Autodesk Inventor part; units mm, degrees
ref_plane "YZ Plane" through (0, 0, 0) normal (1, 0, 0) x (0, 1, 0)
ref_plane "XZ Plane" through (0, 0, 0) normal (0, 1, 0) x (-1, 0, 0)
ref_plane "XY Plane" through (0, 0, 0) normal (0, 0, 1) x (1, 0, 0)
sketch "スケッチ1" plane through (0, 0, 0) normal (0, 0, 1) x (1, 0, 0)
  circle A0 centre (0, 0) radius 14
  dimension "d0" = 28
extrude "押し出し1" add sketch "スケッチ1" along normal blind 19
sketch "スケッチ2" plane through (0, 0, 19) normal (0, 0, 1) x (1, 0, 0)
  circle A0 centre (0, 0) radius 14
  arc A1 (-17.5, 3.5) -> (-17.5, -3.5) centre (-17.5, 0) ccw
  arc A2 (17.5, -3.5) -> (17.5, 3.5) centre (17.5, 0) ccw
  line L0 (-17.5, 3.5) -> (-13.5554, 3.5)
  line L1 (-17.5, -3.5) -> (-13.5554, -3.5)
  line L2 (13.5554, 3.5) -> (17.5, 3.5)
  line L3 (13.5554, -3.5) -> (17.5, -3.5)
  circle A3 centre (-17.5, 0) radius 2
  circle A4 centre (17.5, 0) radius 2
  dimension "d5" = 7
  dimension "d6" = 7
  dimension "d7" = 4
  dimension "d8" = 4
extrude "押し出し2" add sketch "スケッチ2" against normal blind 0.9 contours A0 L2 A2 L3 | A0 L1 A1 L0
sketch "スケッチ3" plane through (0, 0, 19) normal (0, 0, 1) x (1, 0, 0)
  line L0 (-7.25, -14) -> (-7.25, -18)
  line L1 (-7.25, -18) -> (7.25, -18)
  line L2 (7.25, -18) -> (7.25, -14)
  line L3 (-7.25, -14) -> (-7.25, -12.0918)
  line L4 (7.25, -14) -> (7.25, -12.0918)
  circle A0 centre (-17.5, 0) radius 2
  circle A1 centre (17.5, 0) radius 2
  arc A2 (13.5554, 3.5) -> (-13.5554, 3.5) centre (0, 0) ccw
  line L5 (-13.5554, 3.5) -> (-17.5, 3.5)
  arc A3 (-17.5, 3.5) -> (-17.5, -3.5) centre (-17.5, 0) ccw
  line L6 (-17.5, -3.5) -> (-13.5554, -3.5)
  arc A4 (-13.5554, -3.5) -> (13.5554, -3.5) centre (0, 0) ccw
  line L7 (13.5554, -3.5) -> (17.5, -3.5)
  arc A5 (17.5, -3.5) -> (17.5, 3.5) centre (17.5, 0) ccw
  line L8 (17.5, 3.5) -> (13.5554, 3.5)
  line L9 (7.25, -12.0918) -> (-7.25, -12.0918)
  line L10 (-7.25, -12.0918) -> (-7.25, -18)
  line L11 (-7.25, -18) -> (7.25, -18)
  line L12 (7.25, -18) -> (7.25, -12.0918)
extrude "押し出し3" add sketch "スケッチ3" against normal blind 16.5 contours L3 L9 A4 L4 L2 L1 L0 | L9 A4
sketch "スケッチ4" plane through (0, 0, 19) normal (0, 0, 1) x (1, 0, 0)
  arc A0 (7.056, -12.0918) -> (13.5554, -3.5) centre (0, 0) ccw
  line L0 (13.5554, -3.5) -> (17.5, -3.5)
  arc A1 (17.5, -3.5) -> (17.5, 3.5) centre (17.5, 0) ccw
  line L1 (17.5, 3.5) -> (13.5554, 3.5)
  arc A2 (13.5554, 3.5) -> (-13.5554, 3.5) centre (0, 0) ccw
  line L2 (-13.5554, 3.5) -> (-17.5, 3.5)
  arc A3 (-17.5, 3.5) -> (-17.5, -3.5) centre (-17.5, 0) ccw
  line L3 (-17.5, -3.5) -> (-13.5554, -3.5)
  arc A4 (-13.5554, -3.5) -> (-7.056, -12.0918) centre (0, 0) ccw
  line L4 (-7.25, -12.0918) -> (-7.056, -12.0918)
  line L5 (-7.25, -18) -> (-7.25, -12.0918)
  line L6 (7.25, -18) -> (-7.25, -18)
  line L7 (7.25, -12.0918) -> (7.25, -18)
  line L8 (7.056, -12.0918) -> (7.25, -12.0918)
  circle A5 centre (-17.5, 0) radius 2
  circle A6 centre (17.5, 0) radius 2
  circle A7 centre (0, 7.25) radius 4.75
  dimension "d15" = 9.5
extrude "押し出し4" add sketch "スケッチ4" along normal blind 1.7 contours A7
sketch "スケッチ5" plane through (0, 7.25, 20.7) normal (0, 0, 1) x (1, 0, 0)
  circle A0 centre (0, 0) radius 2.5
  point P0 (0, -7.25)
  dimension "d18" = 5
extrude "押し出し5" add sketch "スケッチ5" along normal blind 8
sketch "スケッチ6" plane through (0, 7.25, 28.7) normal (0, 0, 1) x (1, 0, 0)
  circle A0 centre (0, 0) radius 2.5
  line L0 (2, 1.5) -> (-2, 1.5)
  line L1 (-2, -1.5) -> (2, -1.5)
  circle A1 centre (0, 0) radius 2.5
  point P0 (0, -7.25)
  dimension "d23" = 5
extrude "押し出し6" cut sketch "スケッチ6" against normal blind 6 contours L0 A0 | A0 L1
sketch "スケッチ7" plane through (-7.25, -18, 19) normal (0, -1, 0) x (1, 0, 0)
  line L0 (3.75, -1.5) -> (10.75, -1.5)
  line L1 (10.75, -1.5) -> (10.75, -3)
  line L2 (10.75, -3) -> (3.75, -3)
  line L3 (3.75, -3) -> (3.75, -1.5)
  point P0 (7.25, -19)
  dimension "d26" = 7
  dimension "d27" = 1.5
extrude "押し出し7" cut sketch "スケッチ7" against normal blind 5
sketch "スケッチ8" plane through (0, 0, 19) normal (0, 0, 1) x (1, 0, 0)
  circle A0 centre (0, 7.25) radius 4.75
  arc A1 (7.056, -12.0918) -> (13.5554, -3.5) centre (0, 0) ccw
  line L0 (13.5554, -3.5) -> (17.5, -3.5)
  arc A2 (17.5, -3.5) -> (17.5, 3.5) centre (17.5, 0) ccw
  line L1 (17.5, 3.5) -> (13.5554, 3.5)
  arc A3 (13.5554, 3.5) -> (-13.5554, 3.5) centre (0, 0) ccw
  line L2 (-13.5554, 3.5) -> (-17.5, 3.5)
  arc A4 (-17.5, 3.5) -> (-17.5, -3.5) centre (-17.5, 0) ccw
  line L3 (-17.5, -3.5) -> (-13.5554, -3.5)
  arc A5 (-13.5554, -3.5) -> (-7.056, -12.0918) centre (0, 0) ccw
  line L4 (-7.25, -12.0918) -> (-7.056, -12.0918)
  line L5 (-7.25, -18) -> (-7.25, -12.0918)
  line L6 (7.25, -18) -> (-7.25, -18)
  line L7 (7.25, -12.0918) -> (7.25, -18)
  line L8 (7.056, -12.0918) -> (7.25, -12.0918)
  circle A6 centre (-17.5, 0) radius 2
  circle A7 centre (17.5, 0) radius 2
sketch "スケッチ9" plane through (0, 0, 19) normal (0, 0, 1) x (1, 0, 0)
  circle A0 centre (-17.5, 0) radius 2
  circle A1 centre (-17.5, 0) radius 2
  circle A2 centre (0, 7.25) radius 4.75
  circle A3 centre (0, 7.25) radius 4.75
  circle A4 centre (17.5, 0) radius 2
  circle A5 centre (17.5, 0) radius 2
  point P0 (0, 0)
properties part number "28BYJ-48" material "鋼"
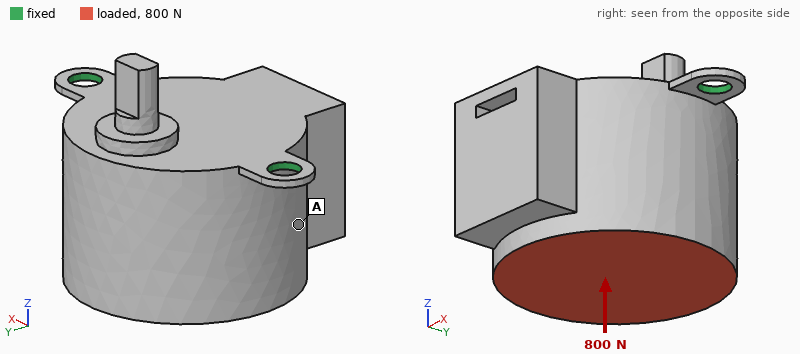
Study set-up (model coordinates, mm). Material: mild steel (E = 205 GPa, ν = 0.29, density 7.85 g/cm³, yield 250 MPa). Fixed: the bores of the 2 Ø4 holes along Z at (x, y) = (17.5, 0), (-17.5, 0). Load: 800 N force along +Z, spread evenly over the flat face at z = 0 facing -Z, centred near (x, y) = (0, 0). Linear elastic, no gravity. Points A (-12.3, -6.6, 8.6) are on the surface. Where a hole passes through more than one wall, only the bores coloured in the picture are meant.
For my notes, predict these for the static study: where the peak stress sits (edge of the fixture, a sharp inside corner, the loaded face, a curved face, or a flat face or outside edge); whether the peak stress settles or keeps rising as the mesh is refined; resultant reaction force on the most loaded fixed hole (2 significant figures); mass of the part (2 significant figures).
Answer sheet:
edge of the fixture
keeps rising
470 N
100 g
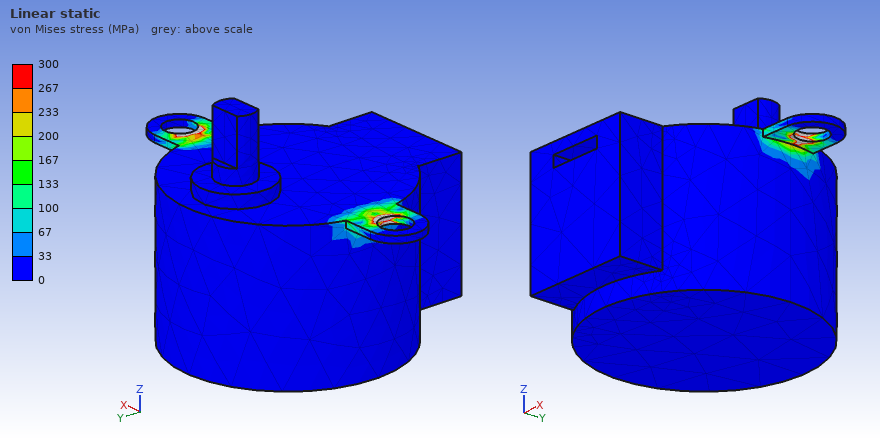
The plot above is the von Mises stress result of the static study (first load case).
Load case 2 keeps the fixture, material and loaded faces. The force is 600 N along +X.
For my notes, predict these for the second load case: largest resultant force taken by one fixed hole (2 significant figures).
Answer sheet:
480 N
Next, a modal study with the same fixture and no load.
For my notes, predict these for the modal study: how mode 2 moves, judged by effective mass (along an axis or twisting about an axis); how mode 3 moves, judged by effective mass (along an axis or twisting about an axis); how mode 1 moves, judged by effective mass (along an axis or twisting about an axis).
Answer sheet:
along Z
along X
along Y
